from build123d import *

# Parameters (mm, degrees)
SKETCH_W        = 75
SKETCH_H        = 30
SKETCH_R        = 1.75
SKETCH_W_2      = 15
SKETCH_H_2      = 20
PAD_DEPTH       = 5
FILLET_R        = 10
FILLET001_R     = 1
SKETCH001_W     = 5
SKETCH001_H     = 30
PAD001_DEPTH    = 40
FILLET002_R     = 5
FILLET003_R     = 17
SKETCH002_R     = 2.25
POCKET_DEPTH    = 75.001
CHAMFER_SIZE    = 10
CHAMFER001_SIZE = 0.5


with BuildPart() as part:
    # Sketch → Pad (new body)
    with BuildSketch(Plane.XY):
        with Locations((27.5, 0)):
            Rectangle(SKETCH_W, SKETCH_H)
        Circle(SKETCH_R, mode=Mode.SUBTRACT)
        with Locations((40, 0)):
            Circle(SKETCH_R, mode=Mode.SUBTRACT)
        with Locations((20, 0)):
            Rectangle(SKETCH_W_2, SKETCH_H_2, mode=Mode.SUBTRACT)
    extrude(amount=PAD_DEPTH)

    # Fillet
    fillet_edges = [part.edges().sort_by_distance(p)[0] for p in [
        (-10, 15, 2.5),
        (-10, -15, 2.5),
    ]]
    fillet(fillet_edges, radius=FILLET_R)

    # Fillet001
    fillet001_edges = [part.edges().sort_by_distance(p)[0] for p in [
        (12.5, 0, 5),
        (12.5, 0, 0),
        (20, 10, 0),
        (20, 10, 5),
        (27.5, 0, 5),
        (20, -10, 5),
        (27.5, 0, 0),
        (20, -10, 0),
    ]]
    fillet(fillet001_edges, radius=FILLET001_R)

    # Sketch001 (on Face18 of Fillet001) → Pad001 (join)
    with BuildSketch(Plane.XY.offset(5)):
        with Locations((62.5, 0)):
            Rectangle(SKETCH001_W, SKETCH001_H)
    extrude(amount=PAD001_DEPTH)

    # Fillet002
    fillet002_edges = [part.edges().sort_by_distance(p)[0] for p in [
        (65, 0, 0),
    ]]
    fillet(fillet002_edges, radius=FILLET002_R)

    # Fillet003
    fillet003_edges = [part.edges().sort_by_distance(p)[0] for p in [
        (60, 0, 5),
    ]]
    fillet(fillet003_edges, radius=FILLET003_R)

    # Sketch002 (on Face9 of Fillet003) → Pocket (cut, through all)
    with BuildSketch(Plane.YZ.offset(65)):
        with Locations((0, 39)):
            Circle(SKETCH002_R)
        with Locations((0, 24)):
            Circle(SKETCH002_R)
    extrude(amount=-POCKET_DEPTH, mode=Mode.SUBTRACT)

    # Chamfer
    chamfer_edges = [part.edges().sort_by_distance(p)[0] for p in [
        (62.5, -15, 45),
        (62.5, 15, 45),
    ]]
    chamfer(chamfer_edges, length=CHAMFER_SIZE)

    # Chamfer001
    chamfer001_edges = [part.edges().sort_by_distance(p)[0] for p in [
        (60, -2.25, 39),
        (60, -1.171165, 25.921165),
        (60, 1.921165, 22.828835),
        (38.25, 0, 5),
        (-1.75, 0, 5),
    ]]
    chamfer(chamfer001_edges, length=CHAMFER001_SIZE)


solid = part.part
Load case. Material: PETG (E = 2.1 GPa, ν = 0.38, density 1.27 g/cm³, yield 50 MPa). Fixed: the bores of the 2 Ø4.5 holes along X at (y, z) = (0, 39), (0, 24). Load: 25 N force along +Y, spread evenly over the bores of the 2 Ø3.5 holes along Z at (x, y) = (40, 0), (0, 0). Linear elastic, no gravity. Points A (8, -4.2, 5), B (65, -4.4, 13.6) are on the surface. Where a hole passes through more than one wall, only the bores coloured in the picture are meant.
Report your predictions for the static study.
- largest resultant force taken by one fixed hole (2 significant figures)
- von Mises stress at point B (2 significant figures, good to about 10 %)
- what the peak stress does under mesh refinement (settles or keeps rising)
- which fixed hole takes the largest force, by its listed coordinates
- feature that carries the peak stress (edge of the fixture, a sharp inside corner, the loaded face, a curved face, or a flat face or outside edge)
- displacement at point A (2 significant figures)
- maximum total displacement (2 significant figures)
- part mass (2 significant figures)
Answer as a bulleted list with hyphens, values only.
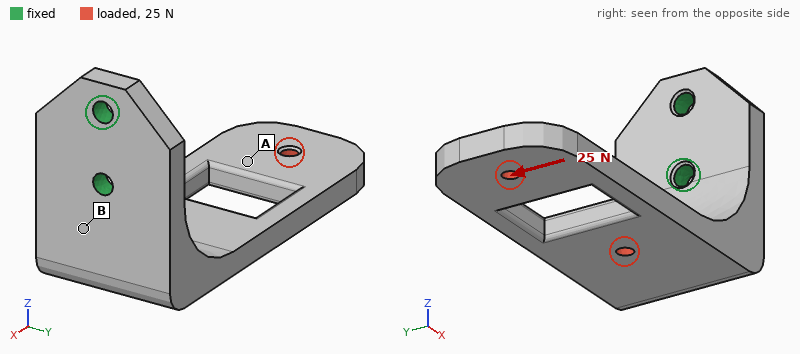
- 50 N
- 2.7 MPa
- keeps rising
- (0, 24)
- edge of the fixture
- 0.71 mm
- 0.93 mm
- 21 g
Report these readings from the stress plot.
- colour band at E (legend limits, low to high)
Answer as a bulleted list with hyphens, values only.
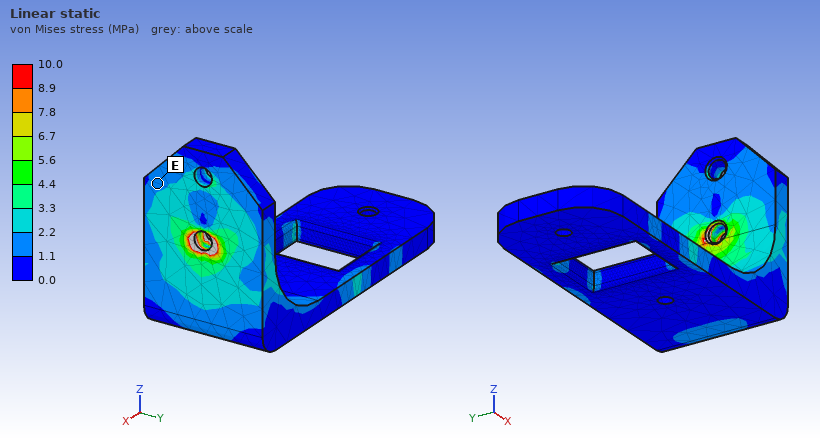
- 1.1 to 2.2 MPa
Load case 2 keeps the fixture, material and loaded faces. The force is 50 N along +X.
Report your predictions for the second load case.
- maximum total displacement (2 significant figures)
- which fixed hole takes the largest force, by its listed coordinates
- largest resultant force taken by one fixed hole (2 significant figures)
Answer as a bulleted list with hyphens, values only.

- 1.0 mm
- (0, 24)
- 77 N
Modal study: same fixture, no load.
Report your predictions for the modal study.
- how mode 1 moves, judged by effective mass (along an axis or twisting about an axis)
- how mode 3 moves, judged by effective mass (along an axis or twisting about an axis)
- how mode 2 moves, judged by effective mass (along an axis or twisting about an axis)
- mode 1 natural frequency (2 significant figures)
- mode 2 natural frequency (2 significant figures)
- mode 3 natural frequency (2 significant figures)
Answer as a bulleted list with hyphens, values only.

- along Z
- along X
- along Y
- 190 Hz
- 320 Hz
- 660 Hz
